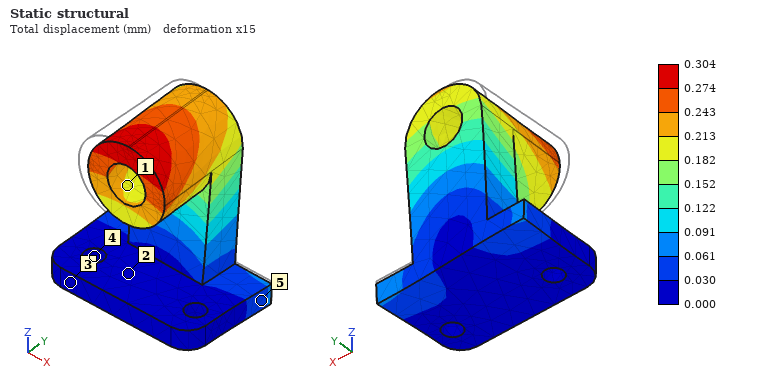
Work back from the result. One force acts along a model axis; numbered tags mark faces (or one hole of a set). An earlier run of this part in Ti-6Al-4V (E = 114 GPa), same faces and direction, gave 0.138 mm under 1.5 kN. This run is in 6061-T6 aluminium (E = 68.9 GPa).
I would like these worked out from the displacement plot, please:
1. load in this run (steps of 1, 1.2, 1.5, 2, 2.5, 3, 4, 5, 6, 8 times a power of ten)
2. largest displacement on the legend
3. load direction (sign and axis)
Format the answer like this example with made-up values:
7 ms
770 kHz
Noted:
2 kN
0.304 mm
+X
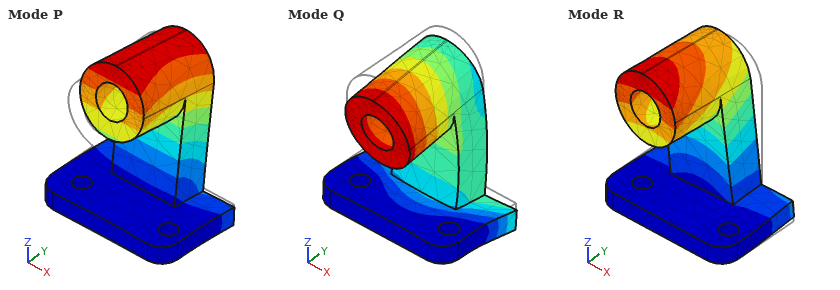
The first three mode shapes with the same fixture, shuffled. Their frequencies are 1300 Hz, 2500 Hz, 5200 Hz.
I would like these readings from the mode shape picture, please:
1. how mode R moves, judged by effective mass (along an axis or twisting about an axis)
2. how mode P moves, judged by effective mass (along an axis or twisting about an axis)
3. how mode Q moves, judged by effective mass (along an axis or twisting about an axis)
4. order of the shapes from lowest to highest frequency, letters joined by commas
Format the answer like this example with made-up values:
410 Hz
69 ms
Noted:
along X
along Y
along Z
P, R, Q
